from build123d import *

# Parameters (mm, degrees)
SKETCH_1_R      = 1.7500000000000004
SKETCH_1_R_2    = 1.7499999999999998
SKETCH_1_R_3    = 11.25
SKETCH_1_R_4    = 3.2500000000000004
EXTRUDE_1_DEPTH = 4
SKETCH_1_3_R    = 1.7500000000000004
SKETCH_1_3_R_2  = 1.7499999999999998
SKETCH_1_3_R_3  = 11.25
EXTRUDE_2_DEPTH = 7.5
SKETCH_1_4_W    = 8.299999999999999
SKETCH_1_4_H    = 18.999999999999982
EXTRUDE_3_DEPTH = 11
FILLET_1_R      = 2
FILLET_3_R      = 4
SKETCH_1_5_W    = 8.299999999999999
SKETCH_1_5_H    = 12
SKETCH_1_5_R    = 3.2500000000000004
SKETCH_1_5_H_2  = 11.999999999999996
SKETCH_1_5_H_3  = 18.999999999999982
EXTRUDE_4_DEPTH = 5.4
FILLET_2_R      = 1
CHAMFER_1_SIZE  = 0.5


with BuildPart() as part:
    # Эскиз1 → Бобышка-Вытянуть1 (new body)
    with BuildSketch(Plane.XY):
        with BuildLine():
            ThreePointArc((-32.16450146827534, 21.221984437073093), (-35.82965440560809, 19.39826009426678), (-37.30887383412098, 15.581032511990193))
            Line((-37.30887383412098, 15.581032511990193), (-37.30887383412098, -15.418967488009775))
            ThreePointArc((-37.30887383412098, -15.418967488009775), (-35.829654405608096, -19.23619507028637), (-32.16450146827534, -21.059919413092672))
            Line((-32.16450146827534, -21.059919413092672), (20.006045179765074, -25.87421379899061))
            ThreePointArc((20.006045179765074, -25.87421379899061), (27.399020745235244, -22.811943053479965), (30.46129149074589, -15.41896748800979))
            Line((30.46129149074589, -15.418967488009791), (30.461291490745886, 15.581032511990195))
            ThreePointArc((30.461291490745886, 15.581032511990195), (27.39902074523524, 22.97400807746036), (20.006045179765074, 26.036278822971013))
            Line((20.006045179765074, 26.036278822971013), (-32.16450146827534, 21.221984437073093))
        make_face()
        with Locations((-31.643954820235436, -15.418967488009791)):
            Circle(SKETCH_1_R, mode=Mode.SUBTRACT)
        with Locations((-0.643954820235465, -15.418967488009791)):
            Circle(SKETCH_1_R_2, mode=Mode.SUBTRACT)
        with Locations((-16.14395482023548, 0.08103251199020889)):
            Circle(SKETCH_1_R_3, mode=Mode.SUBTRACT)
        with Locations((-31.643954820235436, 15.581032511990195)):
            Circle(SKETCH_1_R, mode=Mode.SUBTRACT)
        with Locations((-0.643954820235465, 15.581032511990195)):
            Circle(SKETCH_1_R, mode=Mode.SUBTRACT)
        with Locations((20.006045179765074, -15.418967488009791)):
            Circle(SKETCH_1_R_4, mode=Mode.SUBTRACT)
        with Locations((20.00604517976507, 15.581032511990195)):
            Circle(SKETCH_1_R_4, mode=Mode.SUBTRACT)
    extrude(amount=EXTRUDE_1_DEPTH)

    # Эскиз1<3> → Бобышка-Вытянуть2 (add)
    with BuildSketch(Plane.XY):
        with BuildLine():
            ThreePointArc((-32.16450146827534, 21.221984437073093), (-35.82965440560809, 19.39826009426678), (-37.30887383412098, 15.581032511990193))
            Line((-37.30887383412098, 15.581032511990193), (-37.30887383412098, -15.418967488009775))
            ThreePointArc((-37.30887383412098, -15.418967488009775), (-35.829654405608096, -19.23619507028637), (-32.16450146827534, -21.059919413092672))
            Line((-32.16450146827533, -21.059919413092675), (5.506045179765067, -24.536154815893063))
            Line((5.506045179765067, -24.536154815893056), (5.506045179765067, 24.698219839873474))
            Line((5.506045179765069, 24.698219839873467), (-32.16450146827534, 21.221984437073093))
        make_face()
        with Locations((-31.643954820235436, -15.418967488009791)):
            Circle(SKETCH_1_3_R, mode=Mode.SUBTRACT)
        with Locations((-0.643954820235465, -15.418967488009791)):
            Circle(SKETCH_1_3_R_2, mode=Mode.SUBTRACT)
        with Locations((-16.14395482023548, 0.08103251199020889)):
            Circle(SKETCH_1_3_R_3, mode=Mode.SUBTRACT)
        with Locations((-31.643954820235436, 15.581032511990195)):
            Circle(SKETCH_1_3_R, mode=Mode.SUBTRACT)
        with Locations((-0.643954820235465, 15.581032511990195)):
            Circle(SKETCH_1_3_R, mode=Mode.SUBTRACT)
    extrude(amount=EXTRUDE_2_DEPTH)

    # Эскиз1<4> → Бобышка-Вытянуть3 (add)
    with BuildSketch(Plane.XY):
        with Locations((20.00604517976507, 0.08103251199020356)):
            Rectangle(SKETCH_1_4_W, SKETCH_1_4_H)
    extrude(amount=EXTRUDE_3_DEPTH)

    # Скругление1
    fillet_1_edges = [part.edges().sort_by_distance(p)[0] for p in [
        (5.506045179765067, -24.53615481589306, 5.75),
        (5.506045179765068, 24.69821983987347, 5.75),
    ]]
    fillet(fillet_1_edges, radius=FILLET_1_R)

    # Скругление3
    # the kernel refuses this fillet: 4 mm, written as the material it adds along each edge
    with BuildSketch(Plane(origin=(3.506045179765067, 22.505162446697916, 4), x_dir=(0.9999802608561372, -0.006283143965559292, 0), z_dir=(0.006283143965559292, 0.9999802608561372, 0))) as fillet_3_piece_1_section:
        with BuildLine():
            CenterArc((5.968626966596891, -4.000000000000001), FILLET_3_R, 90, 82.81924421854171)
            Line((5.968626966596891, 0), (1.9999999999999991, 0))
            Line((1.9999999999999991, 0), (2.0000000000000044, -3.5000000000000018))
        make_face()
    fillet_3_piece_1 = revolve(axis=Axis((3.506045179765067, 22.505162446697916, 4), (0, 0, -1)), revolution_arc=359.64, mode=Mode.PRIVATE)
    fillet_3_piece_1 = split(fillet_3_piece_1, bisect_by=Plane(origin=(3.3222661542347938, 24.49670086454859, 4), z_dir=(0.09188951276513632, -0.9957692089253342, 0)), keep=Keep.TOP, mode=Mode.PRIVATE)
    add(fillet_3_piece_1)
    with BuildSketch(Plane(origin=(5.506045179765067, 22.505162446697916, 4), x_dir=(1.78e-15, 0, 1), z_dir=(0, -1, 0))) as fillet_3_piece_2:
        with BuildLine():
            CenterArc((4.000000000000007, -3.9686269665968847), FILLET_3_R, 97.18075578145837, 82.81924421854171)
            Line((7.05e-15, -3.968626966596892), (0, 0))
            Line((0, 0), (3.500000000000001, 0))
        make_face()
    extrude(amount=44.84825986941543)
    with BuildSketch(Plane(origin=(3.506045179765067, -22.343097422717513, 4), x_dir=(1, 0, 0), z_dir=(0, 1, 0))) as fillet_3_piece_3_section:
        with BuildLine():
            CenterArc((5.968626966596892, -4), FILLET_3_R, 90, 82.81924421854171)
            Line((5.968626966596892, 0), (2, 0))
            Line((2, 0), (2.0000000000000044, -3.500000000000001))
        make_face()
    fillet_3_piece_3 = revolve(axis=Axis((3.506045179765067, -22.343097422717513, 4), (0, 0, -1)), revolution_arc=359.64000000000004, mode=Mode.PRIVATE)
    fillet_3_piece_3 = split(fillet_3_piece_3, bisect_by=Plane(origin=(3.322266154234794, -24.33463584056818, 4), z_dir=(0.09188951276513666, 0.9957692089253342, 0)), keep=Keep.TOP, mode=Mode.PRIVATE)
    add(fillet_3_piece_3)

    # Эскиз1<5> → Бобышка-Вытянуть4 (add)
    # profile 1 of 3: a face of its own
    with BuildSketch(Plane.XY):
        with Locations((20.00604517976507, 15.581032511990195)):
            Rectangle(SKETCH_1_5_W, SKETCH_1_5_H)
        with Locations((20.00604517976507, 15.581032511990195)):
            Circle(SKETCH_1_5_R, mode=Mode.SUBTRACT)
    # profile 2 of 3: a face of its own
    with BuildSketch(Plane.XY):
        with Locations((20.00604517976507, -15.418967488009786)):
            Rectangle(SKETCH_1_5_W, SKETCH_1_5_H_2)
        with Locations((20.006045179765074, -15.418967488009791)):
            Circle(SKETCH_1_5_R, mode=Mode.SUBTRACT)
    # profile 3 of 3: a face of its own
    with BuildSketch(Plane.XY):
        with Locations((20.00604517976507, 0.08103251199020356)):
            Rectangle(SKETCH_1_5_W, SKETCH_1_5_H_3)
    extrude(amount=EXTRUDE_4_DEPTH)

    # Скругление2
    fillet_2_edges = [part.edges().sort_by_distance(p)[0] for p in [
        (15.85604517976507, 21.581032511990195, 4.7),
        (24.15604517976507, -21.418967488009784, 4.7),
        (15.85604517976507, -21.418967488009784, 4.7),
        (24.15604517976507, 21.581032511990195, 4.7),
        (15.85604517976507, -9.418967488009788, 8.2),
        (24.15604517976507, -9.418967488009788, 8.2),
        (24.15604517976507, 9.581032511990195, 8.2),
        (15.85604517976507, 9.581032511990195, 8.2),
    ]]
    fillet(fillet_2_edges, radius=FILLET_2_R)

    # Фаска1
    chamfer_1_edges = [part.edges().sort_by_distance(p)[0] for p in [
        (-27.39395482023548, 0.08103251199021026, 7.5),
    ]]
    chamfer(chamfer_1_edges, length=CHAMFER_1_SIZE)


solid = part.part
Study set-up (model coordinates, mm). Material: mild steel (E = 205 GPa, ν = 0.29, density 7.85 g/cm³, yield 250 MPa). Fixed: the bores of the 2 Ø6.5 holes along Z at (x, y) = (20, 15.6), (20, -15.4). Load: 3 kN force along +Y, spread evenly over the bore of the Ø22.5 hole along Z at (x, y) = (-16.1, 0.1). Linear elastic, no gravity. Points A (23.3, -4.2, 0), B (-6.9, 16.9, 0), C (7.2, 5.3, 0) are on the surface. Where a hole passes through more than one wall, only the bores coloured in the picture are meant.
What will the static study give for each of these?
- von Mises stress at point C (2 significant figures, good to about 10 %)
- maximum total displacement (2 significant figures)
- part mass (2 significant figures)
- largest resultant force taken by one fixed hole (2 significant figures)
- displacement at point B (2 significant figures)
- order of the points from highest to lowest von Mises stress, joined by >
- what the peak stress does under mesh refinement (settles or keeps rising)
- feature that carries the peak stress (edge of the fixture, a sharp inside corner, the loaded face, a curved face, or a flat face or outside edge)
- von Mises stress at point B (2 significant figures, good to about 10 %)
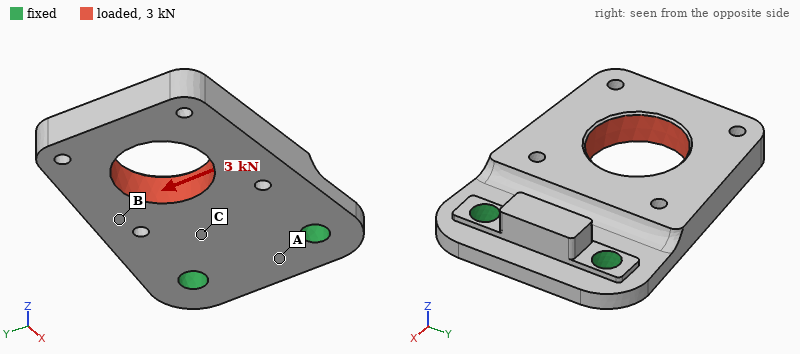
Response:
44 MPa
25 µm
140 g
3.4 kN
10 µm
C > B > A
keeps rising
edge of the fixture
24 MPa
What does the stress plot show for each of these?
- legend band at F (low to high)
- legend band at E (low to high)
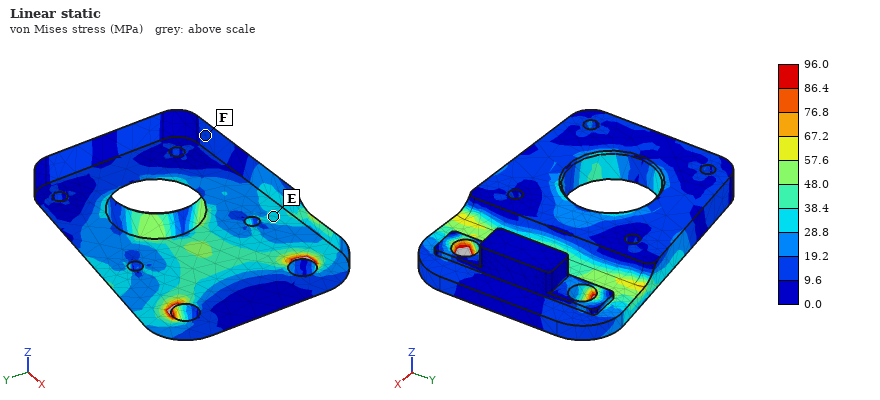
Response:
9.6 to 19.2 MPa
28.8 to 38.4 MPa
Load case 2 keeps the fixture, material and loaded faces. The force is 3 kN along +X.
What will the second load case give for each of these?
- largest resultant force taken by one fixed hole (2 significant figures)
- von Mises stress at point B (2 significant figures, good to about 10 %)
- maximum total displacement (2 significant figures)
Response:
1.5 kN
13 MPa
41 µm
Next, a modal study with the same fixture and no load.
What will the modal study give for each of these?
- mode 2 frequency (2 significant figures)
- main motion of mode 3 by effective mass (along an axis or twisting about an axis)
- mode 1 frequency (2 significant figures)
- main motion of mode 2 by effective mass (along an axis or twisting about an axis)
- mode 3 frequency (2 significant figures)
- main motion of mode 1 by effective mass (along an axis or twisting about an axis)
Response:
4100 Hz
along Y
1200 Hz
twisting about X
7100 Hz
along Z
